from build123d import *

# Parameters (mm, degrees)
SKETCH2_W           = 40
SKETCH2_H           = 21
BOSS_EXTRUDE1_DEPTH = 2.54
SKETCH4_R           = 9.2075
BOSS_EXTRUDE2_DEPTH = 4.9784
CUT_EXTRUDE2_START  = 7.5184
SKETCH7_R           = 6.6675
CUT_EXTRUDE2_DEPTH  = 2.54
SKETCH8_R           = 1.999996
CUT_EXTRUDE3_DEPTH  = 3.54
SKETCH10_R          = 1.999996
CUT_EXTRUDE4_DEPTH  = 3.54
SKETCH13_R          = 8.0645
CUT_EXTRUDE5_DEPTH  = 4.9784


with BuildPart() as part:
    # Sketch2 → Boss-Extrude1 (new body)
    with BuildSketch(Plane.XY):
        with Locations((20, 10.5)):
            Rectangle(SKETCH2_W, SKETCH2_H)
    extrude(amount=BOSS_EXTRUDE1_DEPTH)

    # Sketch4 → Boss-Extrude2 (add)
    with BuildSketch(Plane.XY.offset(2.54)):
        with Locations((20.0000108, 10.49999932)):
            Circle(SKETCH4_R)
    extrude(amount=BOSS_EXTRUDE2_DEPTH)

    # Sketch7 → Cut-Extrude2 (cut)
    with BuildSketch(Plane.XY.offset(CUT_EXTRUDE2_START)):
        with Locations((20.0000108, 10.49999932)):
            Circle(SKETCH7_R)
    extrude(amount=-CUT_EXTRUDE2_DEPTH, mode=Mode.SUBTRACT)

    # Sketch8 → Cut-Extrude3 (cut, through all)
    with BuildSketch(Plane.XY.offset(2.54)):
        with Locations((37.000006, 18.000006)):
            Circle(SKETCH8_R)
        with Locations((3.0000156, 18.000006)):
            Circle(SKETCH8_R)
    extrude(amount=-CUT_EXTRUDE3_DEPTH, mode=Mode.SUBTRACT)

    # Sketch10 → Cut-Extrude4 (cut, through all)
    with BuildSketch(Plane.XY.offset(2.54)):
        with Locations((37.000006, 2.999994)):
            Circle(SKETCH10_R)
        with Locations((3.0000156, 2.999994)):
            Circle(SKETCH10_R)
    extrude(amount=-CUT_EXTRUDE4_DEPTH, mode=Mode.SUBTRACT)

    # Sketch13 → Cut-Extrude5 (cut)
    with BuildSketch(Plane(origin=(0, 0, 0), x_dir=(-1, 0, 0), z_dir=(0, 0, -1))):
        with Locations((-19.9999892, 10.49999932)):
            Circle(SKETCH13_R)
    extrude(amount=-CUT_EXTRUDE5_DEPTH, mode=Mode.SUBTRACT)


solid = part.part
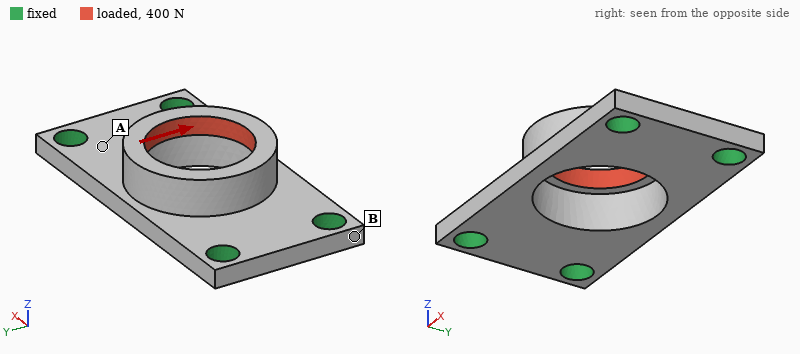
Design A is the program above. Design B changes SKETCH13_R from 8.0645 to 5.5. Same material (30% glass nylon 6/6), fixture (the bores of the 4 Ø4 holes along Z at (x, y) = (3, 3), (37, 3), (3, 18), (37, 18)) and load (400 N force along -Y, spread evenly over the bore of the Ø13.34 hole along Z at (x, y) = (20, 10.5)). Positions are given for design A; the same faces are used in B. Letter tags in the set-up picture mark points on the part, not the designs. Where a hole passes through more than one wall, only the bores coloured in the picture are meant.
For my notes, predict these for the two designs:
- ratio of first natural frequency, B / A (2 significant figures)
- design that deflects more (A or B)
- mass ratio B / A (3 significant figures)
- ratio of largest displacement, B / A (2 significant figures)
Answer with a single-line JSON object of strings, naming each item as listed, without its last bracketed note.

{"ratio of first natural frequency, B / A": "0.92", "design that deflects more": "A", "mass ratio B / A": "1.28", "ratio of largest displacement, B / A": "0.73"}
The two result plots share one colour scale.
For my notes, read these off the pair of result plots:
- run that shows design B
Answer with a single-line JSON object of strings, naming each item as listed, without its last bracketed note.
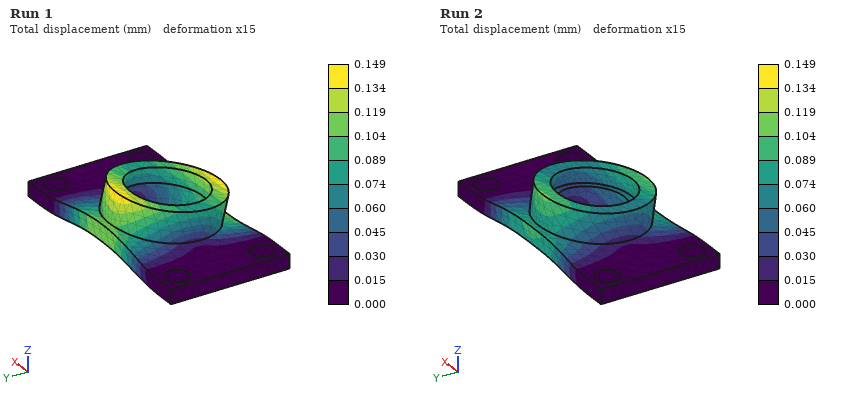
{"run that shows design B": "Run 2"}
